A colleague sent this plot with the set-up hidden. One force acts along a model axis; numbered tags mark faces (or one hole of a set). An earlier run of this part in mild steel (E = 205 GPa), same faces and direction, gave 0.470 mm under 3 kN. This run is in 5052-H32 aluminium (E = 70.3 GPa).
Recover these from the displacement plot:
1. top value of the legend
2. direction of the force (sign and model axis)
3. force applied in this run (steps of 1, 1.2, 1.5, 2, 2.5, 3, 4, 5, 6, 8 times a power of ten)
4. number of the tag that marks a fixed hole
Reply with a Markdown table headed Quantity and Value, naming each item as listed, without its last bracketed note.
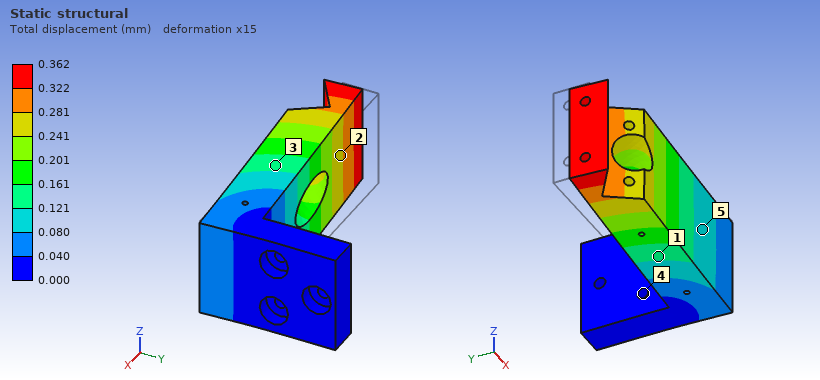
| Quantity | Value |
|---|---|
| top value of the legend | 0.362 mm |
| direction of the force | -Y |
| force applied in this run | 800 N |
| number of the tag that marks a fixed hole | 4 |
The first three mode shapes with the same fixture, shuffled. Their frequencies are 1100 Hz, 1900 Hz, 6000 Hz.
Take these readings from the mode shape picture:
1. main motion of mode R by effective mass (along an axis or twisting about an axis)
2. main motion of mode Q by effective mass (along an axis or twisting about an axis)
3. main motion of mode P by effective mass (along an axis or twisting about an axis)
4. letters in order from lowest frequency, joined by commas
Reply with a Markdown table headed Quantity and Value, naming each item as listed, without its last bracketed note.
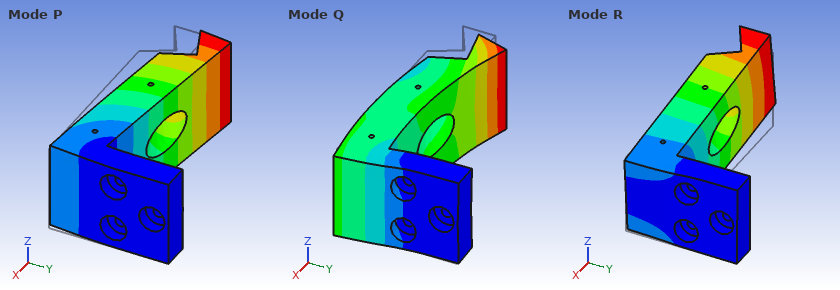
| Quantity | Value |
|---|---|
| main motion of mode R by effective mass | along Z |
| main motion of mode Q by effective mass | along X |
| main motion of mode P by effective mass | along Y |
| letters in order from lowest frequency, joined by commas | P, R, Q |
